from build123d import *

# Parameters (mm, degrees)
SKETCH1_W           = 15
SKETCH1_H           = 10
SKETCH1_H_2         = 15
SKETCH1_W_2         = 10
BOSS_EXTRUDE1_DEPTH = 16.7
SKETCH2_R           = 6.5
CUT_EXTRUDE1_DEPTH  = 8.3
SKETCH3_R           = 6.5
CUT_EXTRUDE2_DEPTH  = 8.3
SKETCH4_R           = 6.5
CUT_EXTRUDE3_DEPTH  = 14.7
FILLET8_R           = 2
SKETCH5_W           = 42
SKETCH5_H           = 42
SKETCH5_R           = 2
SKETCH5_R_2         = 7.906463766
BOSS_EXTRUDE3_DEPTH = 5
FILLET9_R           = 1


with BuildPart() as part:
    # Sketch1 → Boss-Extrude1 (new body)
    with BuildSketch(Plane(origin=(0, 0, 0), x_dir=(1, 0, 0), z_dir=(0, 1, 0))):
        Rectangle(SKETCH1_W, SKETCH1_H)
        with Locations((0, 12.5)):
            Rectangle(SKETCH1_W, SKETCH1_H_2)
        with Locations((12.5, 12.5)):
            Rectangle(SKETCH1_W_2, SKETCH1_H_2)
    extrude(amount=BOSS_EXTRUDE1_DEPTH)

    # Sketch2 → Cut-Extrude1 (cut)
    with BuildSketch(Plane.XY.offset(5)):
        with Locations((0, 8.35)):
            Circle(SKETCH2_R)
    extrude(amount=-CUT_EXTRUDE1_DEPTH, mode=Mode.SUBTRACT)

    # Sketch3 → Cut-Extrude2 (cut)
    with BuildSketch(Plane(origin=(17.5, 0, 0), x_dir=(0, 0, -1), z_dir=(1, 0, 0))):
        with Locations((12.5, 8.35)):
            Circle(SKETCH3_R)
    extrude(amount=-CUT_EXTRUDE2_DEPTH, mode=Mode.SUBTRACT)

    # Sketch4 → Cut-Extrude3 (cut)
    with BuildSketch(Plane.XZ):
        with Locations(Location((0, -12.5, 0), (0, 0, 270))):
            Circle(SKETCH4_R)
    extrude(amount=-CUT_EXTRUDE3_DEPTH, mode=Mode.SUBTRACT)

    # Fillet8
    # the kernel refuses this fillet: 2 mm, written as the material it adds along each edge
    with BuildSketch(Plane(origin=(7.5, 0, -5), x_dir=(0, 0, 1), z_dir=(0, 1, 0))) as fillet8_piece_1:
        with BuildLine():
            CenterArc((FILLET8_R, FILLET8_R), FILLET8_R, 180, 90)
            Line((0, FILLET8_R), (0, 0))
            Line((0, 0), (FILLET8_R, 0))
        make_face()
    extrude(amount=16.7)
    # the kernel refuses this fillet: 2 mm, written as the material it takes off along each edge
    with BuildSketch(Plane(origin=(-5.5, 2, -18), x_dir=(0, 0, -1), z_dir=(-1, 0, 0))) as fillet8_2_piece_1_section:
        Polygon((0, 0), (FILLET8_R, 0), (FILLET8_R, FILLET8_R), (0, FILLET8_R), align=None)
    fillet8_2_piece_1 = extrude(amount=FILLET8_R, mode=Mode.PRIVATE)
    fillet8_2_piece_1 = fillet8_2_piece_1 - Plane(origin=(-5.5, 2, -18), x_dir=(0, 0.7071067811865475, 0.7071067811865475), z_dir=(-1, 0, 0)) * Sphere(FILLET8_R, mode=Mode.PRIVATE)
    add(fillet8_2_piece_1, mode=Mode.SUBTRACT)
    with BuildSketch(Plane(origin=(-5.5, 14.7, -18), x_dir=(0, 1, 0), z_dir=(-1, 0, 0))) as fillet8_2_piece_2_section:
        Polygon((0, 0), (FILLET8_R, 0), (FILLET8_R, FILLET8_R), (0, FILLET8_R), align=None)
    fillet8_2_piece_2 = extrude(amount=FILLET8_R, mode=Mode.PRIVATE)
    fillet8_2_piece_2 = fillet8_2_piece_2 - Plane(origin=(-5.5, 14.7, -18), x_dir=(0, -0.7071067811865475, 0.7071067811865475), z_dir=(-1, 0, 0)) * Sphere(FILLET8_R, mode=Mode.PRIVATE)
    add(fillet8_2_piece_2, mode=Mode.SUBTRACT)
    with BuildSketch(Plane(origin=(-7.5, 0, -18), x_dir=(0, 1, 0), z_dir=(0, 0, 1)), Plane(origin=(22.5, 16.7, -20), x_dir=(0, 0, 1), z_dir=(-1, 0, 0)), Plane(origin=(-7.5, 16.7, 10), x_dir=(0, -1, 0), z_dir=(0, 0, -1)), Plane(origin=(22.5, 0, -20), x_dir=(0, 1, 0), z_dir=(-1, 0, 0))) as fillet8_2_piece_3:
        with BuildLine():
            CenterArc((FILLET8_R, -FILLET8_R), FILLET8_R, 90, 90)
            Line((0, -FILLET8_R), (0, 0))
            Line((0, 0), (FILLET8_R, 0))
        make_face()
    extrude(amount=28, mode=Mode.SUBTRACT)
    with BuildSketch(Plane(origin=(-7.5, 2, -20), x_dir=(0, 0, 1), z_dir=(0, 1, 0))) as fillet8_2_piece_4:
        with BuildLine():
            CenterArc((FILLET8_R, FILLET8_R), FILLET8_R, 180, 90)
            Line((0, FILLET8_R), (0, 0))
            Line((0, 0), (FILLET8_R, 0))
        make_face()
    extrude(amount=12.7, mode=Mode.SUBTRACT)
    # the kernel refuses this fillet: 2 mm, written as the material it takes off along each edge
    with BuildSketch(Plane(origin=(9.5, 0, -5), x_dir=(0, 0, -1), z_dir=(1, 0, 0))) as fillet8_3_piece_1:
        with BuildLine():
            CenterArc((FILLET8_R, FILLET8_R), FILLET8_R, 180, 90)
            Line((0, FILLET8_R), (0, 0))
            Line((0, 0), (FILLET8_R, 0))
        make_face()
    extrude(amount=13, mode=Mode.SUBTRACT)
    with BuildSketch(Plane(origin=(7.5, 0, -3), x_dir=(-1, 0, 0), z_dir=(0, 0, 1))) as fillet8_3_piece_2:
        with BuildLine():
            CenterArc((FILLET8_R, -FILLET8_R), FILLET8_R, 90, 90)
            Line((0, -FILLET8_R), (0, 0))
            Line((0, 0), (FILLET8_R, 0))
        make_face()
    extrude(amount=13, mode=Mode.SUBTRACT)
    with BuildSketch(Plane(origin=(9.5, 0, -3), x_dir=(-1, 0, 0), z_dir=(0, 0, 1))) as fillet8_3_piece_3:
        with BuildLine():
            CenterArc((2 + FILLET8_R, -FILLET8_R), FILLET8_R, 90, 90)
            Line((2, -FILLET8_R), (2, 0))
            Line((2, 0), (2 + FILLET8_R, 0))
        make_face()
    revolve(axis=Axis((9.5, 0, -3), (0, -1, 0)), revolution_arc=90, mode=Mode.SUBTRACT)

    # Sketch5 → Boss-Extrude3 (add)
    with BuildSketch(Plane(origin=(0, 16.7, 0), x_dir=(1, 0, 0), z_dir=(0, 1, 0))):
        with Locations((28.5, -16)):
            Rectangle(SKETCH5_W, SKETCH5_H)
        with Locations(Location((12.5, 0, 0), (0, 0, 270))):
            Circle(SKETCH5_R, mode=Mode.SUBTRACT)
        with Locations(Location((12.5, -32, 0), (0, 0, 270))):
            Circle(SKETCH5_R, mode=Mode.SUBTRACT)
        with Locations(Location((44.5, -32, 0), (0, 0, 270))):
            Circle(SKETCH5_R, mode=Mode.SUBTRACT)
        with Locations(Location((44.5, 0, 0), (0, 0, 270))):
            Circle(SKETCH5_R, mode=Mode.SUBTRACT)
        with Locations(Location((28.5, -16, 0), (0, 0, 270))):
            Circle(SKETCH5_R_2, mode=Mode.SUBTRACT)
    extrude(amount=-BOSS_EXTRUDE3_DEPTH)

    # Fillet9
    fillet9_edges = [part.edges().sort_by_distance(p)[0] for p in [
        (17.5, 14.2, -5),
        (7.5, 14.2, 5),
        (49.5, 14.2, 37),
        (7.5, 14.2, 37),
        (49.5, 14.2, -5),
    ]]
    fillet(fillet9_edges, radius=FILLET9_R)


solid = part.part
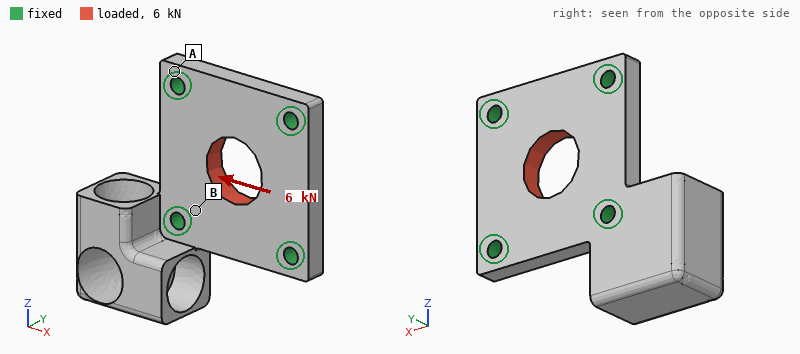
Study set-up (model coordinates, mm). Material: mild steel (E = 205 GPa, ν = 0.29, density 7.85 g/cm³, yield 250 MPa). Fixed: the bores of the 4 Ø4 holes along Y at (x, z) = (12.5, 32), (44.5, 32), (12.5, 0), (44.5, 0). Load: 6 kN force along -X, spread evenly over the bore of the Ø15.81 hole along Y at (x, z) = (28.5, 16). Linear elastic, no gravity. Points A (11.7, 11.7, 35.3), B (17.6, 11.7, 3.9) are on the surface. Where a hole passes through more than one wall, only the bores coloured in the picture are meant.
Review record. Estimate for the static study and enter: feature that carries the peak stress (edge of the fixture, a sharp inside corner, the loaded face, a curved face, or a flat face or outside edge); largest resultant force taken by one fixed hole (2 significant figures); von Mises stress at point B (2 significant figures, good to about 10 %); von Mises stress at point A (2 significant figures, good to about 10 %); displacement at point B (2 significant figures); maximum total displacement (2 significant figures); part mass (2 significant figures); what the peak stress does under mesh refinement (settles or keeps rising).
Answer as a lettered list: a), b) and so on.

a) edge of the fixture
b) 1.7 kN
c) 30 MPa
d) 10.0 MPa
e) 0.98 µm
f) 3.3 µm
g) 95 g
h) keeps rising
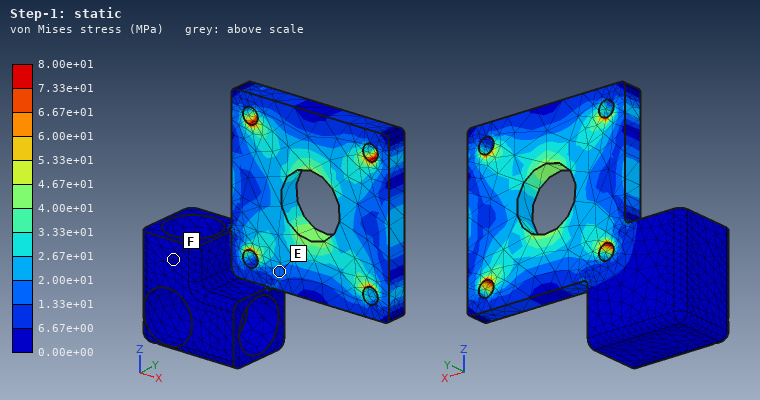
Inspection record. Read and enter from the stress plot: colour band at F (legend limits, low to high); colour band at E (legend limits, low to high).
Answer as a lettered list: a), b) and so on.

a) 0.00e+00 to 6.67e+00 MPa
b) 1.33e+01 to 2.00e+01 MPa
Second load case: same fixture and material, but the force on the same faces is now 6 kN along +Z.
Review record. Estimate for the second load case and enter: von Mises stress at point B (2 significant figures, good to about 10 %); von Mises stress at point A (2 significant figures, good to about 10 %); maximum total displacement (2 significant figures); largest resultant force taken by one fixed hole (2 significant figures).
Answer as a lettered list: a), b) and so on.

a) 30 MPa
b) 15 MPa
c) 3.4 µm
d) 1.7 kN
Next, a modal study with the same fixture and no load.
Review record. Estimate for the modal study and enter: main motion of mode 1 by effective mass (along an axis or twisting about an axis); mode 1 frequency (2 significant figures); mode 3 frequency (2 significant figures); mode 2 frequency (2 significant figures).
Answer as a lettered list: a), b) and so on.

a) along Y
b) 4500 Hz
c) 9400 Hz
d) 6700 Hz
